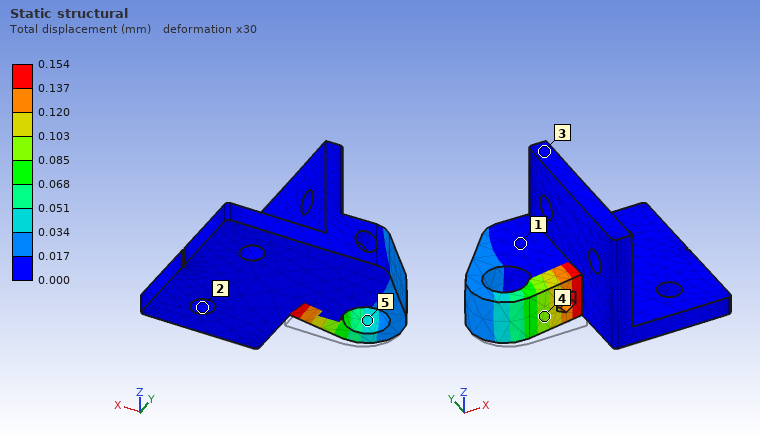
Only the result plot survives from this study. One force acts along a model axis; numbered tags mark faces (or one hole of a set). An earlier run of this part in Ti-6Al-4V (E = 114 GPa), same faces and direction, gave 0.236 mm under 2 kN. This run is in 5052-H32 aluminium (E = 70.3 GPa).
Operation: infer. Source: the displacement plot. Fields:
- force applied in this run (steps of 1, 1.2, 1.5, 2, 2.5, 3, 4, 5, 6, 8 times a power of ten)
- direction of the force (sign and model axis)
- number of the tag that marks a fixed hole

800 N
+Y
2
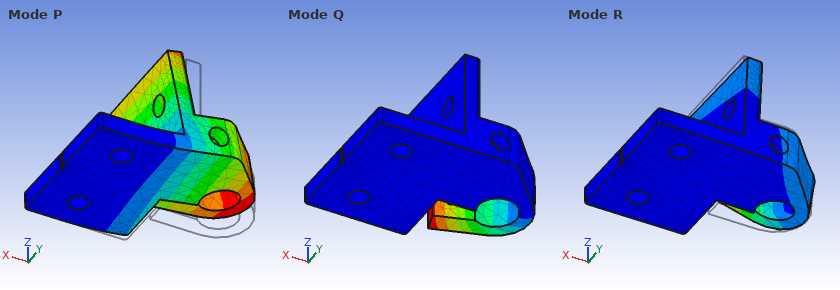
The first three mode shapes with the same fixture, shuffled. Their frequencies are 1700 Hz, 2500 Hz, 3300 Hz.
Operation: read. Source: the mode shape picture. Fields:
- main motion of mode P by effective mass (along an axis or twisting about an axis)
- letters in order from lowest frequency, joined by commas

along Z
P, Q, R
